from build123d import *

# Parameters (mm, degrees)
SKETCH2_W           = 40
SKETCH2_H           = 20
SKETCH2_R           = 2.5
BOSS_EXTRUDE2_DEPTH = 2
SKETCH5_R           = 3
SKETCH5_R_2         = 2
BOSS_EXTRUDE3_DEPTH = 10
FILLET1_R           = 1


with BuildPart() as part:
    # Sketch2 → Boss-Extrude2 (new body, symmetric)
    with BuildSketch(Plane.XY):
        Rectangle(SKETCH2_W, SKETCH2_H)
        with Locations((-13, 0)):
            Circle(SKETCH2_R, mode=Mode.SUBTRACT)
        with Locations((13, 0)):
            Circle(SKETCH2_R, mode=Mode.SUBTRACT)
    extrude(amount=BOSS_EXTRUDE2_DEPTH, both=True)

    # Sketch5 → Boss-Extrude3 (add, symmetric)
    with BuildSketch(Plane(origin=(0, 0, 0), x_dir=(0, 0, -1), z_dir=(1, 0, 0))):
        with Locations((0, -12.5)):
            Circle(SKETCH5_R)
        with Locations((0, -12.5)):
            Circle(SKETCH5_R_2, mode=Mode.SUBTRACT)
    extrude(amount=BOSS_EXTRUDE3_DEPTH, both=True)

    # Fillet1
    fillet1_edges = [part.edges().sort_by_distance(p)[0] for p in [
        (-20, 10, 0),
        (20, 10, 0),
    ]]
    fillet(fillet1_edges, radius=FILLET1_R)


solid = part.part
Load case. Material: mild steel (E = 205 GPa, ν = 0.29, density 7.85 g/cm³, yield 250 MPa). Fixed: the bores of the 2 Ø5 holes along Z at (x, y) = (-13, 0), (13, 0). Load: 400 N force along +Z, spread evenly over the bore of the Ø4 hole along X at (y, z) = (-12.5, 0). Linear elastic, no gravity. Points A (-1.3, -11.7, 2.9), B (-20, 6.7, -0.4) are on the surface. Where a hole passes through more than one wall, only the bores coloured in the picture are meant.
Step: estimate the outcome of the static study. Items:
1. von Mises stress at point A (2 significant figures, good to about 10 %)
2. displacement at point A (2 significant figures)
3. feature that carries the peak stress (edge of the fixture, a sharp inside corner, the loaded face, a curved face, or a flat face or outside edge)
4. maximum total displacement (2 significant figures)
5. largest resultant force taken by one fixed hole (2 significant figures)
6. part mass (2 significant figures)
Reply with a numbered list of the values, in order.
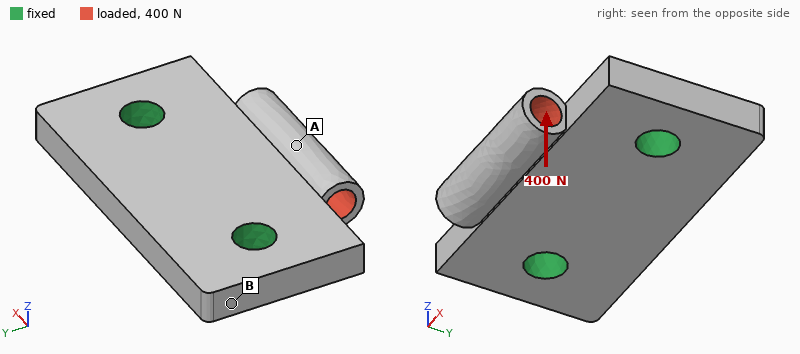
1. 27 MPa
2. 12 µm
3. the loaded face
4. 17 µm
5. 200 N
6. 26 g
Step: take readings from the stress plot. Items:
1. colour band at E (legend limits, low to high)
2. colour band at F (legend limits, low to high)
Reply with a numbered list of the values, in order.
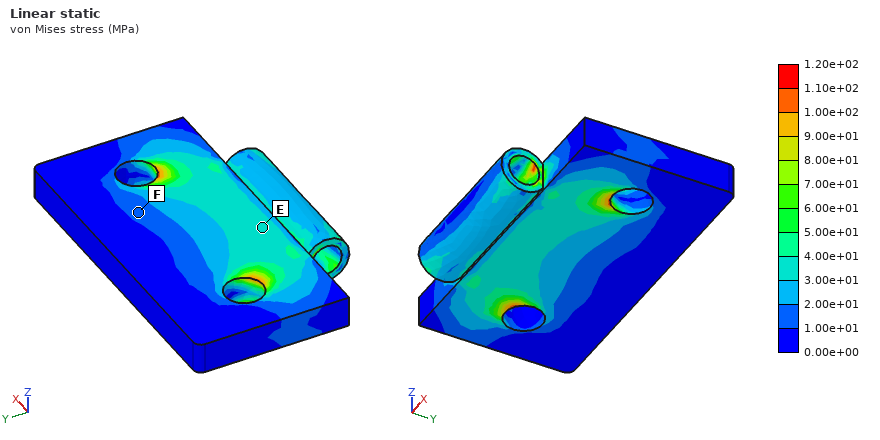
1. 3.00e+01 to 4.00e+01 MPa
2. 1.00e+01 to 2.00e+01 MPa
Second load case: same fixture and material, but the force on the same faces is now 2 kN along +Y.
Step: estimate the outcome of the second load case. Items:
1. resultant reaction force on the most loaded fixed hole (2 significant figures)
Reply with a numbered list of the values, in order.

1. 1.0 kN
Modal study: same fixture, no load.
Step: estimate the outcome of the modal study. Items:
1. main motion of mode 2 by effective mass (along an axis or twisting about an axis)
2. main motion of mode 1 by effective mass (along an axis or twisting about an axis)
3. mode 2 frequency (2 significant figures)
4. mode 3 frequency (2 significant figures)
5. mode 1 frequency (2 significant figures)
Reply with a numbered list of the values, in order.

1. along Z
2. along Z
3. 26 kHz
4. 34 kHz
5. 16 kHz
